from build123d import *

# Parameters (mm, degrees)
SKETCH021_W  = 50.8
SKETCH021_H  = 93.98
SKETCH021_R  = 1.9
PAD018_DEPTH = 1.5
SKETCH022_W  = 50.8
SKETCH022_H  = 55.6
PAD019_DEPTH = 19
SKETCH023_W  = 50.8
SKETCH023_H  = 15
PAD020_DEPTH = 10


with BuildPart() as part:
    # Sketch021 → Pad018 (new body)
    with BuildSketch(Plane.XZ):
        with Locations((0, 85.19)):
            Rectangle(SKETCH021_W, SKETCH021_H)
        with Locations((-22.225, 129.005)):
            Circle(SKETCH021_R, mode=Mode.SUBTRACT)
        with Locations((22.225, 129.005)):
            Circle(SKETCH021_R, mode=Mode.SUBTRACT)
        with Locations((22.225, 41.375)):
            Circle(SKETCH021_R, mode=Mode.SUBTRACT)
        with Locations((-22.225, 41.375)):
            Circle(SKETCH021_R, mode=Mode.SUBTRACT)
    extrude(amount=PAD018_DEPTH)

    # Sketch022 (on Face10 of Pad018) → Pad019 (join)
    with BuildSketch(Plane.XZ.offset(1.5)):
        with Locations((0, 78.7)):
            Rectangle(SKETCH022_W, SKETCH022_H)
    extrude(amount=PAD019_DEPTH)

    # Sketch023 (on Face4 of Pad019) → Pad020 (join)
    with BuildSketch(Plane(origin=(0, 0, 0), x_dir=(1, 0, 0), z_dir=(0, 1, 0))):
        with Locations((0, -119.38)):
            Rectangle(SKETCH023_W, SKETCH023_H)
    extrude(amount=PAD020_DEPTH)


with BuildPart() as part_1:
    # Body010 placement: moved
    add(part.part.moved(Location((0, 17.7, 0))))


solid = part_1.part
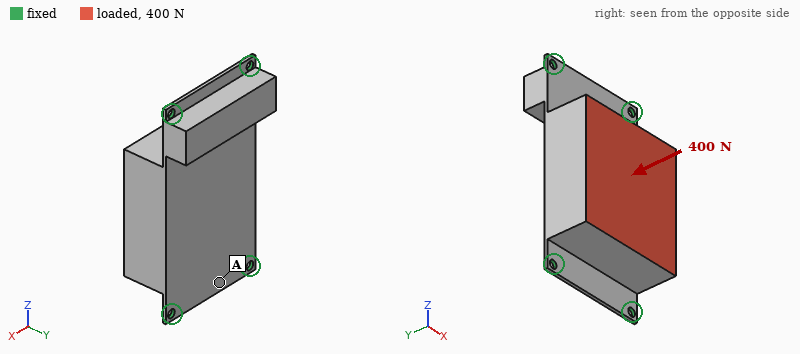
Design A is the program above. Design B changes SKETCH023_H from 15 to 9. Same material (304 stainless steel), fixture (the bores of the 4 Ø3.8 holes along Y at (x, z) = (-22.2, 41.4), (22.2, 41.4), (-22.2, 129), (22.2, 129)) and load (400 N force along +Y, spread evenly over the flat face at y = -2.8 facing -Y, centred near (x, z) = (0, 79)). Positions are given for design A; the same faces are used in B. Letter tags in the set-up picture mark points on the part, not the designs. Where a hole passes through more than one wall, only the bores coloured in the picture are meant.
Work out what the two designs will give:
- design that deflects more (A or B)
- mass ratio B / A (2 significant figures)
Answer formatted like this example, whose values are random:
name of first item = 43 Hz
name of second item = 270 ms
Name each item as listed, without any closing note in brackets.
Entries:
design that deflects more = B
mass ratio B / A = 0.96
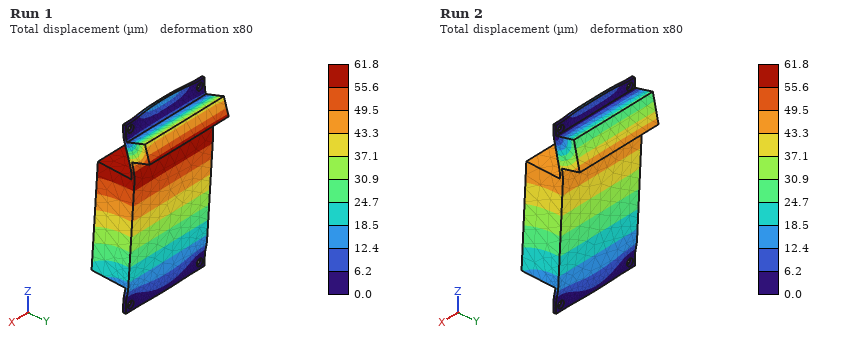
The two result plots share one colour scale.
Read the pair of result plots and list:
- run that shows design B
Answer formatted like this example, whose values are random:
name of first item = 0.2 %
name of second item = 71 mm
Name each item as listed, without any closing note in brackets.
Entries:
run that shows design B = Run 1
